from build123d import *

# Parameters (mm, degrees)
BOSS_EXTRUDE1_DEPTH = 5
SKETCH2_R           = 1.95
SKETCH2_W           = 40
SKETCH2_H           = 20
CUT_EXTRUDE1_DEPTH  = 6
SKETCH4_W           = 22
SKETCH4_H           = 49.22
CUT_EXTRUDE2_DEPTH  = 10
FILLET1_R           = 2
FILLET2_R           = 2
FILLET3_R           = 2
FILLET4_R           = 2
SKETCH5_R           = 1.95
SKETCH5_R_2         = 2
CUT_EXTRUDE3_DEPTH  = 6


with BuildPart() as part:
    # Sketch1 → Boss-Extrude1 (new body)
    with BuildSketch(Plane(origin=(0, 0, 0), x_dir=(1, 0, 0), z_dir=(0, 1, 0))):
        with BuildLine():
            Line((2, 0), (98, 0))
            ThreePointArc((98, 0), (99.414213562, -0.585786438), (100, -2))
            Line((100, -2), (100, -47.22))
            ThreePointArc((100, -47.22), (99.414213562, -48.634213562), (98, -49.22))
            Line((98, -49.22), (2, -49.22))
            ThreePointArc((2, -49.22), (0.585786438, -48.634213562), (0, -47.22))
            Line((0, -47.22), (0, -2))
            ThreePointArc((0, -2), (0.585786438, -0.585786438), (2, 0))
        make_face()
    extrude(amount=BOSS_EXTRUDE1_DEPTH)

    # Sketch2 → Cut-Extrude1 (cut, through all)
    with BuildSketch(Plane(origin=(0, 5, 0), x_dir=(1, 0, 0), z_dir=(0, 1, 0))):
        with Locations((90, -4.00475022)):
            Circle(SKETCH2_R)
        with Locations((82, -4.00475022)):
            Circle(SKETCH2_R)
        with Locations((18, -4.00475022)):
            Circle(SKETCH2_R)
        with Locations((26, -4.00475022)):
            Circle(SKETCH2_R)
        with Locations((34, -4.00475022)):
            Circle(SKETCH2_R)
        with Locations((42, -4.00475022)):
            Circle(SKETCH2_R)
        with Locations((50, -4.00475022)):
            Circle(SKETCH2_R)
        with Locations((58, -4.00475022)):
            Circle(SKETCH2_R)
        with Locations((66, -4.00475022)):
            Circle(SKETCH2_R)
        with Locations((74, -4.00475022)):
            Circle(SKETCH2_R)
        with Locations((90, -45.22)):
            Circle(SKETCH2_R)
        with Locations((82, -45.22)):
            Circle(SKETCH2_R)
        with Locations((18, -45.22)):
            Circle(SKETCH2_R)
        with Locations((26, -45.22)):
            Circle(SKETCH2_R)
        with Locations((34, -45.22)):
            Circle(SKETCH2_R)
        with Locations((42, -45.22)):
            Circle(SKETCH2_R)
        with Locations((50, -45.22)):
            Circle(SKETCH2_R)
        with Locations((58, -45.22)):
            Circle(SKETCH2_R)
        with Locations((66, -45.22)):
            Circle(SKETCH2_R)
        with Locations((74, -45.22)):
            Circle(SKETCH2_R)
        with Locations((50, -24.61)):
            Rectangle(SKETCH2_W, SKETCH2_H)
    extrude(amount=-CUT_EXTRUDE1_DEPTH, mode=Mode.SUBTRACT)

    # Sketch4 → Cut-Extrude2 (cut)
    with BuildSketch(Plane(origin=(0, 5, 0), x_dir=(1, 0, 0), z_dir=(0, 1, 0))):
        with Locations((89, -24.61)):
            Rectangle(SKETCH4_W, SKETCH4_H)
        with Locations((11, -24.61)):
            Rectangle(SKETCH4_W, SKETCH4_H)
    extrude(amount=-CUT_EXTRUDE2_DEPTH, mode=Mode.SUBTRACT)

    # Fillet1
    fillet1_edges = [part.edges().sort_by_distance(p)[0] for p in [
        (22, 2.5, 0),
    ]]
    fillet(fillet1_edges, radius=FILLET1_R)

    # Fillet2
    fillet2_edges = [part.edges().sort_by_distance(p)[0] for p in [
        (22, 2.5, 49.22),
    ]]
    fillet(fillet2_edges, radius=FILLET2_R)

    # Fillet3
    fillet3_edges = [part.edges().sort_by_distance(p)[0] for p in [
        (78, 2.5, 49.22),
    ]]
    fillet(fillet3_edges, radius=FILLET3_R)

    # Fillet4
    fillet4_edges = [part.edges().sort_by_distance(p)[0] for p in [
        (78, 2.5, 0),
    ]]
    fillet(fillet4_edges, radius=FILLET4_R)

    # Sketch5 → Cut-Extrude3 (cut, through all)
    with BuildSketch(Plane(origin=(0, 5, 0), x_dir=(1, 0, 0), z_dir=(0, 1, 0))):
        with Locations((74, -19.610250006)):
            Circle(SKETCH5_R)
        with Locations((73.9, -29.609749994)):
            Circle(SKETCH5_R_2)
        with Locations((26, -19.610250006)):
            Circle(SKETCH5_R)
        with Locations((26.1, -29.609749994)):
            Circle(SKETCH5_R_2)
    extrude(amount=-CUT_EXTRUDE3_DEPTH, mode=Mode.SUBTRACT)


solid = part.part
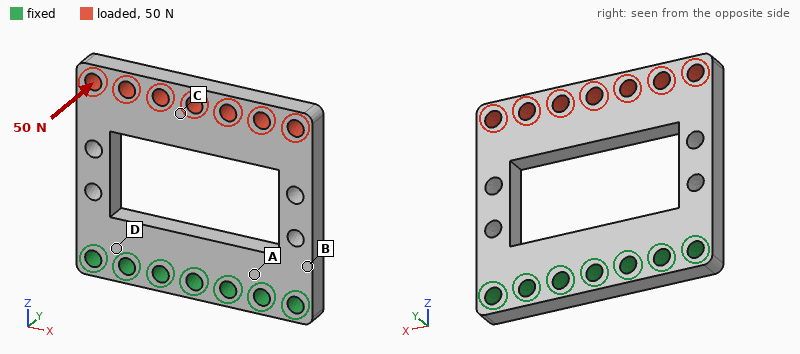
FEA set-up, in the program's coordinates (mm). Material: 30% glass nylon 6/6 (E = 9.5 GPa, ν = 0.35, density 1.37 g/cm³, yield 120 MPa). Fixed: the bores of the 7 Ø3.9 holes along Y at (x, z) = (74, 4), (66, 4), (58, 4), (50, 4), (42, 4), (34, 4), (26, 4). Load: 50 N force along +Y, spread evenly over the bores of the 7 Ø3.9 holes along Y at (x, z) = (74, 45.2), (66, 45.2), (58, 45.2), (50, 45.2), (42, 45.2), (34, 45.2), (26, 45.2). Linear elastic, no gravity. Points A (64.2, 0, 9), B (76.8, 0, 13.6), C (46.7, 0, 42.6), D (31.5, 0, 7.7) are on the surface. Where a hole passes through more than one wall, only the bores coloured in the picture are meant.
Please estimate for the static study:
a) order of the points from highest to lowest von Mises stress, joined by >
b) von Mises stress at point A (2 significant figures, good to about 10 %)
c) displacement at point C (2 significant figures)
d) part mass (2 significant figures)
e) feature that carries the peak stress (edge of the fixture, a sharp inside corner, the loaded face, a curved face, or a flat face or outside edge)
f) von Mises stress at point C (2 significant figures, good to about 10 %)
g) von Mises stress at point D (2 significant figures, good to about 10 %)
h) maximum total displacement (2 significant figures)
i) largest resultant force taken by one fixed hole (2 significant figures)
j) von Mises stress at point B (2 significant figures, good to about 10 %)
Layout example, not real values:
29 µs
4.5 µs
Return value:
B > D > A > C
6.5 MPa
0.66 mm
12 g
a curved face
3.4 MPa
11 MPa
0.85 mm
19 N
20 MPa
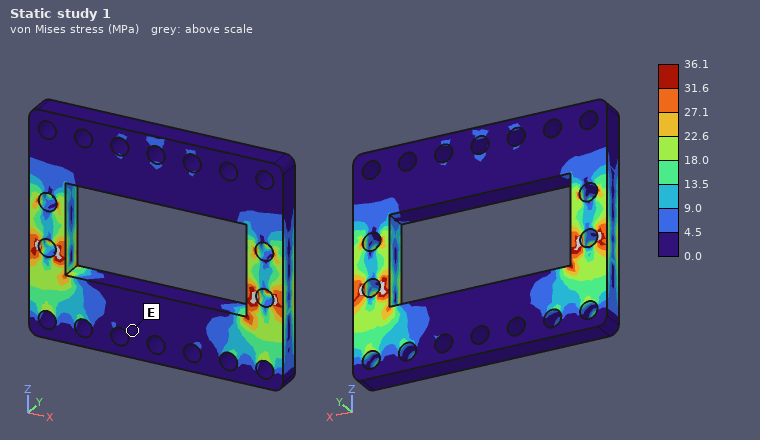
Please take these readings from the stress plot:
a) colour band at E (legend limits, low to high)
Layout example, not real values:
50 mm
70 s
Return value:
0.0 to 4.5 MPa
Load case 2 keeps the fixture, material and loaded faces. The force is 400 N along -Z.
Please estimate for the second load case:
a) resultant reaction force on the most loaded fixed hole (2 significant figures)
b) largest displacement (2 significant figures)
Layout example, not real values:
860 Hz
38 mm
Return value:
190 N
66 µm
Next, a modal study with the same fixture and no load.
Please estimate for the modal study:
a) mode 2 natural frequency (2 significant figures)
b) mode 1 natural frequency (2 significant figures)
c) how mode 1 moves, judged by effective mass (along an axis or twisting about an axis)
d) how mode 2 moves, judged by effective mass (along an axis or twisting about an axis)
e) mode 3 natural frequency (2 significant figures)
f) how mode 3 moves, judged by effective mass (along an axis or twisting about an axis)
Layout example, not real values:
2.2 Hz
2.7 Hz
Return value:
1600 Hz
670 Hz
along Y
twisting about Z
2400 Hz
along X
